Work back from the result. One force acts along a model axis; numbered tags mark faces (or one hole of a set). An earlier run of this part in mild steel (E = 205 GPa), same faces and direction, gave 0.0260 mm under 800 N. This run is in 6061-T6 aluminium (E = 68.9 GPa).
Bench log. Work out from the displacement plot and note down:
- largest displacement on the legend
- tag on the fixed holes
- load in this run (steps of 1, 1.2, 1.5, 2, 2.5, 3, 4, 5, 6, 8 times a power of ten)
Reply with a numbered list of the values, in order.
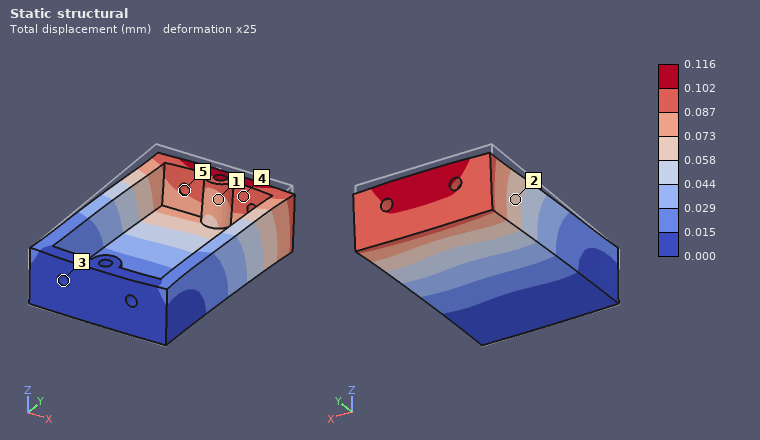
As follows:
1. 0.116 mm
2. 3
3. 1.2 kN
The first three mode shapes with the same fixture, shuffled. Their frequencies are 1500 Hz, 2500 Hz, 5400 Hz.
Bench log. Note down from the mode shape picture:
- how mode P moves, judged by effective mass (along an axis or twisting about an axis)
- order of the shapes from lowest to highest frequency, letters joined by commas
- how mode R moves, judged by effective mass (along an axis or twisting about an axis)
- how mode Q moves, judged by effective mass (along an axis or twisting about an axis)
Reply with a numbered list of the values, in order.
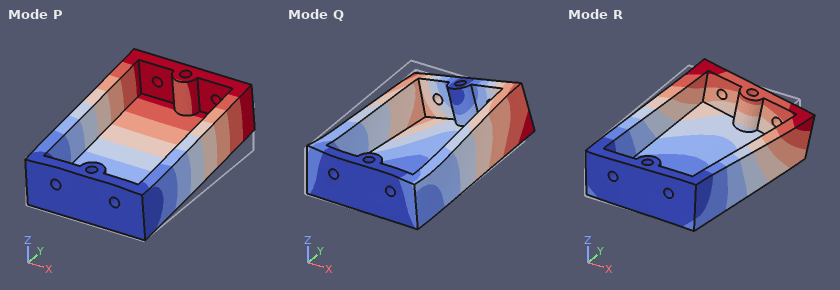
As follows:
1. along Z
2. P, R, Q
3. along X
4. along X
